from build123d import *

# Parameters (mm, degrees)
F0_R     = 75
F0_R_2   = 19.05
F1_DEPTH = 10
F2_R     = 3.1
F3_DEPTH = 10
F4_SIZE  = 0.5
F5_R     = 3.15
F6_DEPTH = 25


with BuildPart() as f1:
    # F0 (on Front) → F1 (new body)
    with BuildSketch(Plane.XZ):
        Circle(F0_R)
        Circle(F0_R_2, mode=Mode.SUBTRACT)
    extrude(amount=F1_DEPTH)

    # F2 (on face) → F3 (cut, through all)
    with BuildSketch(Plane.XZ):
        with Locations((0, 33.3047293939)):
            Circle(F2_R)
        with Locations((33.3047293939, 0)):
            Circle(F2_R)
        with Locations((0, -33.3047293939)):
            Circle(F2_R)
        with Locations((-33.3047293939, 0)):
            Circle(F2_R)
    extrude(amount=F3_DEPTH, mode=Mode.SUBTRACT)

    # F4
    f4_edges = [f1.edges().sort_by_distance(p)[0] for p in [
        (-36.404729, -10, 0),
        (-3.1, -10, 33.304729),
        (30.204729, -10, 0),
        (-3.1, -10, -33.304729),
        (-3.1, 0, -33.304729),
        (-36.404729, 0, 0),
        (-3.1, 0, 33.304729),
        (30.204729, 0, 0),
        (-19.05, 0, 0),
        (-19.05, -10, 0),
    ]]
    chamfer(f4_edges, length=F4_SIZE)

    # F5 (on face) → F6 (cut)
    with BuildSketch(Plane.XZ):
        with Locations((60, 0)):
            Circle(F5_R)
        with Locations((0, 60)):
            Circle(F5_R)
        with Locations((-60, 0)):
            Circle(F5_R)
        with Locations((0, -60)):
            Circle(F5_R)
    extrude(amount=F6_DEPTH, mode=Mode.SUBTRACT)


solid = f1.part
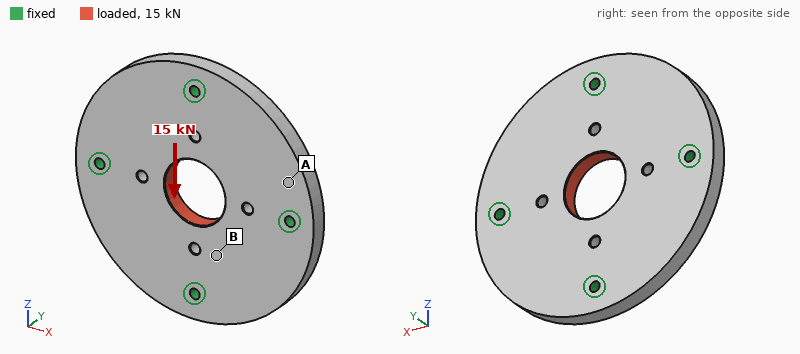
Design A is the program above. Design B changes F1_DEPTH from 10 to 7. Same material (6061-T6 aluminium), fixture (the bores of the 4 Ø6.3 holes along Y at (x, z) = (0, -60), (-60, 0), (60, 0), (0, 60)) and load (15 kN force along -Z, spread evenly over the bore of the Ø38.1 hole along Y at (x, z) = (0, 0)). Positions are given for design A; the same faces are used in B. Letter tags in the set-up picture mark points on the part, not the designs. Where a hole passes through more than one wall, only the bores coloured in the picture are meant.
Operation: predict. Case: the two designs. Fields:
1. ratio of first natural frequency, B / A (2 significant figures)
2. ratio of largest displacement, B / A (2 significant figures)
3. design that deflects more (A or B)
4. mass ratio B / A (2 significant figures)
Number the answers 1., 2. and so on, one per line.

1. 0.76
2. 1.4
3. B
4. 0.70
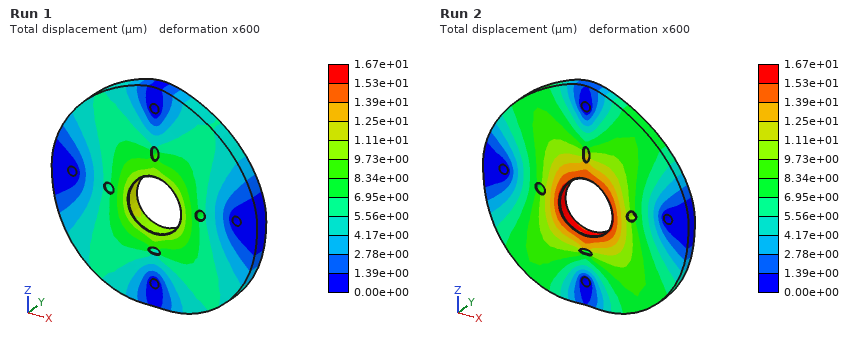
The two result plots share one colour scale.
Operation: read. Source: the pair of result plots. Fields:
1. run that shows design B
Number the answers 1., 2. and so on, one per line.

1. Run 2
